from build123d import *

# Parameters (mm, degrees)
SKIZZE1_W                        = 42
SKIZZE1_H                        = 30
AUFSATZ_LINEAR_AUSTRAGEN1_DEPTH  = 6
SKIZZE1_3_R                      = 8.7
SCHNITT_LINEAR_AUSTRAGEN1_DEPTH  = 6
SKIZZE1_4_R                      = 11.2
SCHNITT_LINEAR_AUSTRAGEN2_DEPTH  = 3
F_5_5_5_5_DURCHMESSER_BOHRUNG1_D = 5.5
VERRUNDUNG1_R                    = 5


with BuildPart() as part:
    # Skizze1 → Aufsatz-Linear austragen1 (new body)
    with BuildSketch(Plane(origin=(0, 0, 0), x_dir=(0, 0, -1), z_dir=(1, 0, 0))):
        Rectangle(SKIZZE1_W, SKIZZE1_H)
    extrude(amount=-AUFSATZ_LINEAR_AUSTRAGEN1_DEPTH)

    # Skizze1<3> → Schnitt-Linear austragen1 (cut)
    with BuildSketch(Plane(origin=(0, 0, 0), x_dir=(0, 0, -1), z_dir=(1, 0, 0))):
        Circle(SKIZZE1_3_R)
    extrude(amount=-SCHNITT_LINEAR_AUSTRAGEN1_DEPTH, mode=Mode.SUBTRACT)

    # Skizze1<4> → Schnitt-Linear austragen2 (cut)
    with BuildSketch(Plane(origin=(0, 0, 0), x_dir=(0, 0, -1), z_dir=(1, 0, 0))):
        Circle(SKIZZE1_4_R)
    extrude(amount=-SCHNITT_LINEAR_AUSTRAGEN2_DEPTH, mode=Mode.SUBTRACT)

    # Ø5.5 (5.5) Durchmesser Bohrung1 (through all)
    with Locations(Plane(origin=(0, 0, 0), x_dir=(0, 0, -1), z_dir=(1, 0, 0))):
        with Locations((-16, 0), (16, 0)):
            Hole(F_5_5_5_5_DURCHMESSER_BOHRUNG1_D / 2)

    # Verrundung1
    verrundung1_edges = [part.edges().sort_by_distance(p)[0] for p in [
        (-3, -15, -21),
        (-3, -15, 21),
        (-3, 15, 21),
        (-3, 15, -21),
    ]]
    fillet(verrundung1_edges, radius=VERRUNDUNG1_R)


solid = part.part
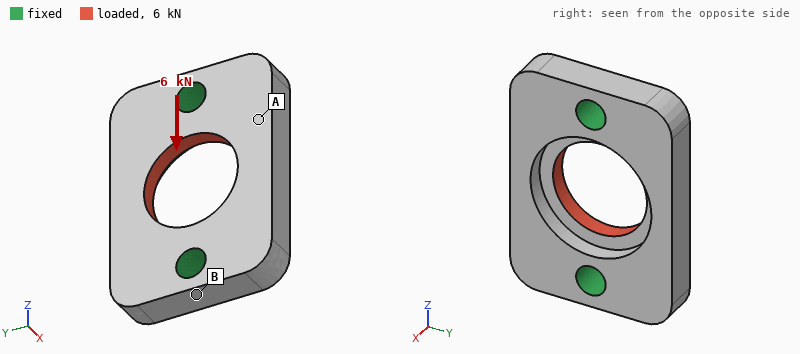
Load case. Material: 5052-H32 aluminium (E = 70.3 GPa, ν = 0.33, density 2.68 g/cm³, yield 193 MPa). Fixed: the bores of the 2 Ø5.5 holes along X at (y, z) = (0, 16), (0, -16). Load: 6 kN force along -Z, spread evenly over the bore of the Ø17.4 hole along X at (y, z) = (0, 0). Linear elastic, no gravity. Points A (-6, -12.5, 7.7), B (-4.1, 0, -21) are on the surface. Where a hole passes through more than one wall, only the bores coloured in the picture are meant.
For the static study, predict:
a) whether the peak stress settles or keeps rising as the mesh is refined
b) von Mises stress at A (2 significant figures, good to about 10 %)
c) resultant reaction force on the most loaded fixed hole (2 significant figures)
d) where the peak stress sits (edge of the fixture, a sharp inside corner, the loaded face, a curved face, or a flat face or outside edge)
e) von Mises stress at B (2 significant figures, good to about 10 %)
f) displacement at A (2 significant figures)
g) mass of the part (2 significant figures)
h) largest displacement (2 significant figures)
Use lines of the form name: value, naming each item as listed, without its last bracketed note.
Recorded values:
whether the peak stress settles or keeps rising as the mesh is refined: keeps rising
von Mises stress at A: 10 MPa
resultant reaction force on the most loaded fixed hole: 3.0 kN
where the peak stress sits: edge of the fixture
von Mises stress at B: 39 MPa
displacement at A: 11 µm
mass of the part: 14 g
largest displacement: 14 µm
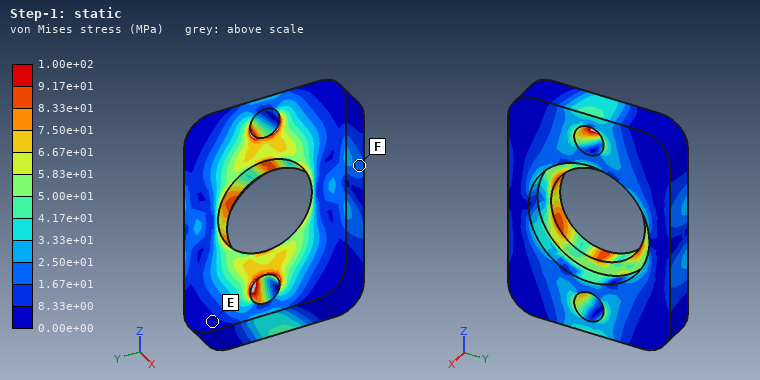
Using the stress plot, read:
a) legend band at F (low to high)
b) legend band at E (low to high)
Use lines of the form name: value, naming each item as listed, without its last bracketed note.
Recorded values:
legend band at F: 1.67e+01 to 2.50e+01 MPa
legend band at E: 0.00e+00 to 8.33e+00 MPa
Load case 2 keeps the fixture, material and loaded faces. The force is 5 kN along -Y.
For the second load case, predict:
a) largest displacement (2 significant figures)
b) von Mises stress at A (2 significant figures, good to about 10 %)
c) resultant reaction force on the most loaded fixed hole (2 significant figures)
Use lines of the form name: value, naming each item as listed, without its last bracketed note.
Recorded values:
largest displacement: 20 µm
von Mises stress at A: 38 MPa
resultant reaction force on the most loaded fixed hole: 2.5 kN
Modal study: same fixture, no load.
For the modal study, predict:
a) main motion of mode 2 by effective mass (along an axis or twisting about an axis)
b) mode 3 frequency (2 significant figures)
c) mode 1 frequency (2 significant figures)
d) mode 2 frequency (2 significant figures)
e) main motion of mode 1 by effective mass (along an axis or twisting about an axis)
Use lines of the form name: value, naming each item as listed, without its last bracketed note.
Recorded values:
main motion of mode 2 by effective mass: along X
mode 3 frequency: 26 kHz
mode 1 frequency: 16 kHz
mode 2 frequency: 17 kHz
main motion of mode 1 by effective mass: twisting about Z
